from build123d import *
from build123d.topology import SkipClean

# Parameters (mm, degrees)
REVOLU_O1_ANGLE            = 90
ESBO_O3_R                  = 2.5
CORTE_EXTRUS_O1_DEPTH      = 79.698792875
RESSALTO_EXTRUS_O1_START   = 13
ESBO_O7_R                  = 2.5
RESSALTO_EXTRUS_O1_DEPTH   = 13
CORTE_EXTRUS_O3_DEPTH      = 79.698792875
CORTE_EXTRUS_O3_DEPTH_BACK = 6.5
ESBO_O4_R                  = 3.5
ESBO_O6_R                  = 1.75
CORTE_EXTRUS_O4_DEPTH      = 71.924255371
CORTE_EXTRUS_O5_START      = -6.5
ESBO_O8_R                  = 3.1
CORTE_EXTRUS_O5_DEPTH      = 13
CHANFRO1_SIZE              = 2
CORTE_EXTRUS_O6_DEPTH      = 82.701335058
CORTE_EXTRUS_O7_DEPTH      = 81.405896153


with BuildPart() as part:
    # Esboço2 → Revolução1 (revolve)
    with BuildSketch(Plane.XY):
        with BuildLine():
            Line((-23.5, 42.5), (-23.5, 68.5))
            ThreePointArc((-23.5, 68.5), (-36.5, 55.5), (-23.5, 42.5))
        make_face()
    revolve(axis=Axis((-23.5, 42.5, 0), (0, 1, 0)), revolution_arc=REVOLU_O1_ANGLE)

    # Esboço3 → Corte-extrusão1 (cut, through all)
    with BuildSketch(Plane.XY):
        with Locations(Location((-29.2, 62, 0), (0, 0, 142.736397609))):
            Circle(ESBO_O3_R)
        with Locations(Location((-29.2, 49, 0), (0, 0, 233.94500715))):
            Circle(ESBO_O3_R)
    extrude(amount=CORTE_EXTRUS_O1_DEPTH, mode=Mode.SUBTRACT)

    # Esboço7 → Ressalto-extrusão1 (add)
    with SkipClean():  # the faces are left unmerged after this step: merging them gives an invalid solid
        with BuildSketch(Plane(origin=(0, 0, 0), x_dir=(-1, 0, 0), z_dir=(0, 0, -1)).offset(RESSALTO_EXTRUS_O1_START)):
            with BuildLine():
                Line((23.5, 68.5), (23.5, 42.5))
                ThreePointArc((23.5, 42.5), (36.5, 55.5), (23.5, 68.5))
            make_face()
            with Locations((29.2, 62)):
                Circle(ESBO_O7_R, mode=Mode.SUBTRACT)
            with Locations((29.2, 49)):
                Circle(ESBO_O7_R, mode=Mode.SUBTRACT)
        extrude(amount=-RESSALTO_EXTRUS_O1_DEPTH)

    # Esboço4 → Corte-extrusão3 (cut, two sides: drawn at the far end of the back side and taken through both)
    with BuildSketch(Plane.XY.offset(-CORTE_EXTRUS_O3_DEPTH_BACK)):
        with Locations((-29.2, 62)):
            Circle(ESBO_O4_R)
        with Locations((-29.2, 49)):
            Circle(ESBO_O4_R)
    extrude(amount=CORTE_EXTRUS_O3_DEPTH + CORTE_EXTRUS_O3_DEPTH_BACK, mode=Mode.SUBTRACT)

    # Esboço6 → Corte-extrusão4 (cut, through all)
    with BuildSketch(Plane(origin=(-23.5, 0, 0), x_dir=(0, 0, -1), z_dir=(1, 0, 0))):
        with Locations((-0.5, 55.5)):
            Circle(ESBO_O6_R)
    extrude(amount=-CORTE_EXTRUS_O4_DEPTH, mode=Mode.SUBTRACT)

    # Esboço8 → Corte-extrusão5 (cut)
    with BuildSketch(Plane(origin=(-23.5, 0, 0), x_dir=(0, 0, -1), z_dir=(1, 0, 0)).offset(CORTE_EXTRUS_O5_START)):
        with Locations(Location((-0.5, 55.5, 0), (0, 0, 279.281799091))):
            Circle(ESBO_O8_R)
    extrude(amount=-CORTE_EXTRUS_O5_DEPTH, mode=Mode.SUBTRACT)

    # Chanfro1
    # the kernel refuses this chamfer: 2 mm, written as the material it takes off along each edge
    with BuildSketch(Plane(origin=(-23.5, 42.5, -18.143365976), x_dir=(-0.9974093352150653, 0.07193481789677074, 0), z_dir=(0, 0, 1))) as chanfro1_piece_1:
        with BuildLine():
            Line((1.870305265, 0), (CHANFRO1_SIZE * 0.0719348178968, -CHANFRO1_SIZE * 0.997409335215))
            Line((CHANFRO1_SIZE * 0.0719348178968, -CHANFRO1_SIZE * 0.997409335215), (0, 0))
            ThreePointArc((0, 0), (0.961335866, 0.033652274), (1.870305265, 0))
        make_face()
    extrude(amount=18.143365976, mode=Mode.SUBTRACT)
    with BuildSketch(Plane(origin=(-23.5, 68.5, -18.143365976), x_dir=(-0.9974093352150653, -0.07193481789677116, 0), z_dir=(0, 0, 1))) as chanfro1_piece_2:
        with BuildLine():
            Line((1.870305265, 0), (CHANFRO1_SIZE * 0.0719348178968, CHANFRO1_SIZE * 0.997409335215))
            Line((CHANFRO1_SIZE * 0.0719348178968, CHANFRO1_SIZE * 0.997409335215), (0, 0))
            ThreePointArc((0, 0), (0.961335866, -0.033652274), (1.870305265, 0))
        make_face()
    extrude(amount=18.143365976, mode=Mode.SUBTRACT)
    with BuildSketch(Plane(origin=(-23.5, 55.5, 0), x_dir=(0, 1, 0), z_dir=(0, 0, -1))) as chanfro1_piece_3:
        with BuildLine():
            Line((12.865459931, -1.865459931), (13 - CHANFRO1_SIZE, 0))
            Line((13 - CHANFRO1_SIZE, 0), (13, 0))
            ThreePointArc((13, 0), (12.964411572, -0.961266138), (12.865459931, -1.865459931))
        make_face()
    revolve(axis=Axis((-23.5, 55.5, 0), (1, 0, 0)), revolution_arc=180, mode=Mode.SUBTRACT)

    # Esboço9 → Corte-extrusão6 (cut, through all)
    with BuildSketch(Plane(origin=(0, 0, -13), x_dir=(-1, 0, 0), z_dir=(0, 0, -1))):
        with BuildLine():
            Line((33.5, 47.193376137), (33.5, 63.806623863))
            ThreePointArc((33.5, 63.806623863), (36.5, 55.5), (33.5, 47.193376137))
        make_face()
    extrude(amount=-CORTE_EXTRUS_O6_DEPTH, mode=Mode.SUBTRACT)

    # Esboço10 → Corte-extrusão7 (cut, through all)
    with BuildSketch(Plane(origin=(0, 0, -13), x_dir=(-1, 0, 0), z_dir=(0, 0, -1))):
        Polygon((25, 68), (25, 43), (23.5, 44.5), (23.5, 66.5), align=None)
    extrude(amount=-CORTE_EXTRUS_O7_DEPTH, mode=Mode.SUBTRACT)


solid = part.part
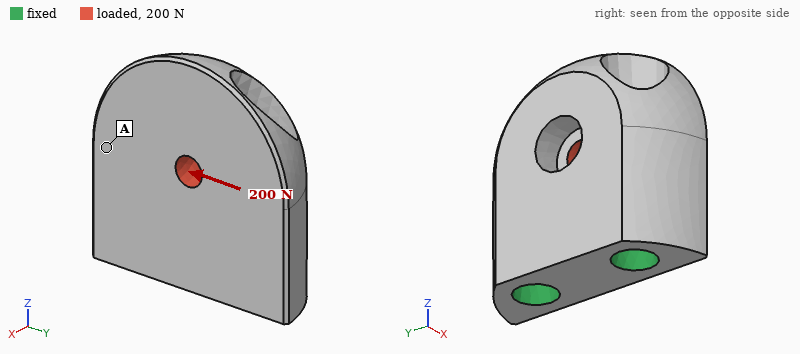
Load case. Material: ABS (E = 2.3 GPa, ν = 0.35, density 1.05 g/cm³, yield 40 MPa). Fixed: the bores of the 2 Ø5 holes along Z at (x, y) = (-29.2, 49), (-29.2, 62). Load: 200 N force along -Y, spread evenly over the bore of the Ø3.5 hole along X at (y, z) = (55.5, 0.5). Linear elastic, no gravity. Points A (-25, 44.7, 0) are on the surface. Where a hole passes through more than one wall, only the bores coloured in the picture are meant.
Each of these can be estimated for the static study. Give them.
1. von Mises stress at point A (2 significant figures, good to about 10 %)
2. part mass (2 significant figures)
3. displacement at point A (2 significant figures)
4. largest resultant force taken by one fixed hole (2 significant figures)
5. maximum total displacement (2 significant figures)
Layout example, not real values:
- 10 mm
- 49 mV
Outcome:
- 1.8 MPa
- 2.7 g
- 36 µm
- 150 N
- 56 µm
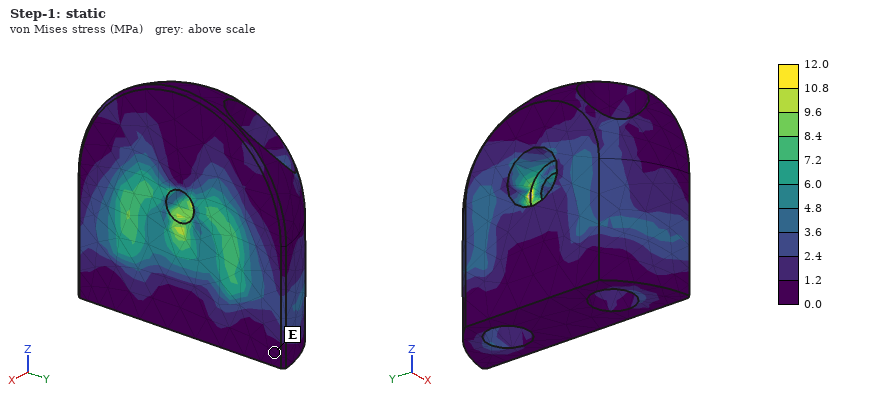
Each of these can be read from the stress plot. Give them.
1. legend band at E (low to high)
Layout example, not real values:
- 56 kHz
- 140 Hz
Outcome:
- 0.0 to 1.2 MPa
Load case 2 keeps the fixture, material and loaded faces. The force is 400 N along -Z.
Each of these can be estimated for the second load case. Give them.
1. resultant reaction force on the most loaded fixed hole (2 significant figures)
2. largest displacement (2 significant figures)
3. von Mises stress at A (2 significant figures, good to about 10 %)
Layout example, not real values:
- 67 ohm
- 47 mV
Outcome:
- 210 N
- 81 µm
- 2.0 MPa
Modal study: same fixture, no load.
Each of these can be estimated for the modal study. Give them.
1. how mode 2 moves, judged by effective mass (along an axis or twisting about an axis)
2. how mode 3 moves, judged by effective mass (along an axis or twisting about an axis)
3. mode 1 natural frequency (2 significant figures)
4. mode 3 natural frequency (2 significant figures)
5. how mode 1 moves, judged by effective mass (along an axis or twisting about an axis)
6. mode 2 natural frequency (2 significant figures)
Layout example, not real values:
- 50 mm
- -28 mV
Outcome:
- along Y
- twisting about Z
- 4400 Hz
- 9700 Hz
- along X
- 7700 Hz
